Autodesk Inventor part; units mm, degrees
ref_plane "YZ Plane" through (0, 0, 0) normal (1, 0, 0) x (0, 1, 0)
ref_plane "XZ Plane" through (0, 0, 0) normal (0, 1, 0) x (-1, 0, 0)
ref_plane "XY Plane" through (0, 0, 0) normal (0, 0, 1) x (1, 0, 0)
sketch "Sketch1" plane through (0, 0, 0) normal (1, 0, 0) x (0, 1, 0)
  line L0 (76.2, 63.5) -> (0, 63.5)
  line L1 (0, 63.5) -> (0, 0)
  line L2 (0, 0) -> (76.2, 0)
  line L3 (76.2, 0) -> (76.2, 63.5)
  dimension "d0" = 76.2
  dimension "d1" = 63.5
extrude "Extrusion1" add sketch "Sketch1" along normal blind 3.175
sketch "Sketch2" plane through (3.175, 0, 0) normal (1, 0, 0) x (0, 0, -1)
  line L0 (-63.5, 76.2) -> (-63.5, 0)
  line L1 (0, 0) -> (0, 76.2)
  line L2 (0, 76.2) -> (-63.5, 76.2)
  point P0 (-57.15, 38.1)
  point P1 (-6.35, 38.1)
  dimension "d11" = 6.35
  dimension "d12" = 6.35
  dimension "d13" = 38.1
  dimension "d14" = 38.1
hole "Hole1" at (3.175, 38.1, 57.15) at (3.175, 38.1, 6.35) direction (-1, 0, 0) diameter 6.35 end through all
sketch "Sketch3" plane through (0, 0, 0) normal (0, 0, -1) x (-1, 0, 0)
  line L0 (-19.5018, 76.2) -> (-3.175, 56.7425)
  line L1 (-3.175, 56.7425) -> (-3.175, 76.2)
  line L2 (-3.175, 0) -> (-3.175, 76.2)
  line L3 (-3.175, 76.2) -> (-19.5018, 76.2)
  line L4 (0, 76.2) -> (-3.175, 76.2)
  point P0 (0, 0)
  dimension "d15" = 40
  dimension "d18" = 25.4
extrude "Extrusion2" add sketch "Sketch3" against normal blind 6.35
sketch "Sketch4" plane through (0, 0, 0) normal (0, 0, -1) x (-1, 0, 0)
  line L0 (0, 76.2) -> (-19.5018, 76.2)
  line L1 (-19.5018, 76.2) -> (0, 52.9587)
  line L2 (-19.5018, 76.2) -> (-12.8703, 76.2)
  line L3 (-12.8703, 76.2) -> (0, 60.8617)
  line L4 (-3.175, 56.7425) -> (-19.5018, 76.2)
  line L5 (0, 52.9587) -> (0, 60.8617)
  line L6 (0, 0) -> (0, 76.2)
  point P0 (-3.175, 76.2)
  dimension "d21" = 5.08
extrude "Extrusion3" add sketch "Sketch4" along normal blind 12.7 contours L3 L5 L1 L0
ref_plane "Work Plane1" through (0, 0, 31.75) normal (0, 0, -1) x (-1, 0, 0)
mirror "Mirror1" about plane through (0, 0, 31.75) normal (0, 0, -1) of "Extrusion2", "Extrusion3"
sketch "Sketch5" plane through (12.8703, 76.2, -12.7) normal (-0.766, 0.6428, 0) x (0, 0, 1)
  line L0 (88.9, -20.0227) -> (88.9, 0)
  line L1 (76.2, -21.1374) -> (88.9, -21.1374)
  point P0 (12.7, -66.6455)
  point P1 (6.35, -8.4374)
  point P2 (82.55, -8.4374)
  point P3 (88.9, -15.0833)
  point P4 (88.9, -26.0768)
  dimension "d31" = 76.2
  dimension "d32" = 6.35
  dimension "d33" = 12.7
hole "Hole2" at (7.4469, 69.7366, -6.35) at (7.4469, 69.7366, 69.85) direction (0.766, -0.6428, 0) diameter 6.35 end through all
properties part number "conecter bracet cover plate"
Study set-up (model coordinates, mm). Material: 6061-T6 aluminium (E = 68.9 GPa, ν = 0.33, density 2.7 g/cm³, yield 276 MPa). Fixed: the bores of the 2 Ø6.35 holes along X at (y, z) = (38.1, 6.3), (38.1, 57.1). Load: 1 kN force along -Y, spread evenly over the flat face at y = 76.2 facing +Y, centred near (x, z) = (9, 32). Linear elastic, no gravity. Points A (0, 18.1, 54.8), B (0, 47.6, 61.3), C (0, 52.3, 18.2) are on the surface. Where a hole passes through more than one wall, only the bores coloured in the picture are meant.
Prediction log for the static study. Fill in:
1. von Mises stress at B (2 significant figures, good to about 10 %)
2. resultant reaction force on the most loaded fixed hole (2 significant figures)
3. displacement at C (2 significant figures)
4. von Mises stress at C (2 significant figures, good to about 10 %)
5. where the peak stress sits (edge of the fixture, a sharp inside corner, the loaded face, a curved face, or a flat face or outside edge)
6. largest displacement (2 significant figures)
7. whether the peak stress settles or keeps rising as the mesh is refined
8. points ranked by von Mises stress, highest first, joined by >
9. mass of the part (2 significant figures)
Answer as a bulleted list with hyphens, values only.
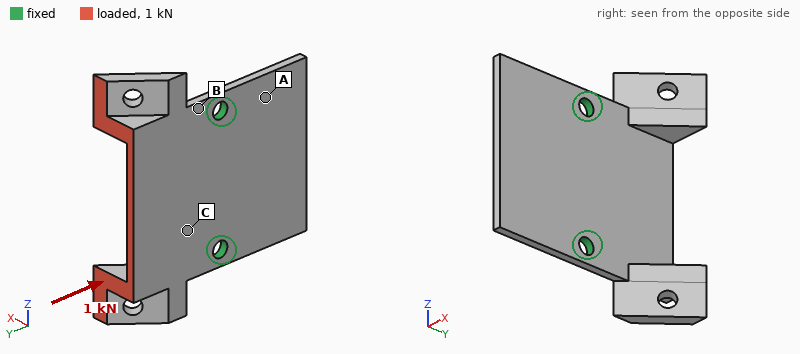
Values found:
- 91 MPa
- 500 N
- 0.087 mm
- 56 MPa
- edge of the fixture
- 0.53 mm
- keeps rising
- B > C > A
- 54 g
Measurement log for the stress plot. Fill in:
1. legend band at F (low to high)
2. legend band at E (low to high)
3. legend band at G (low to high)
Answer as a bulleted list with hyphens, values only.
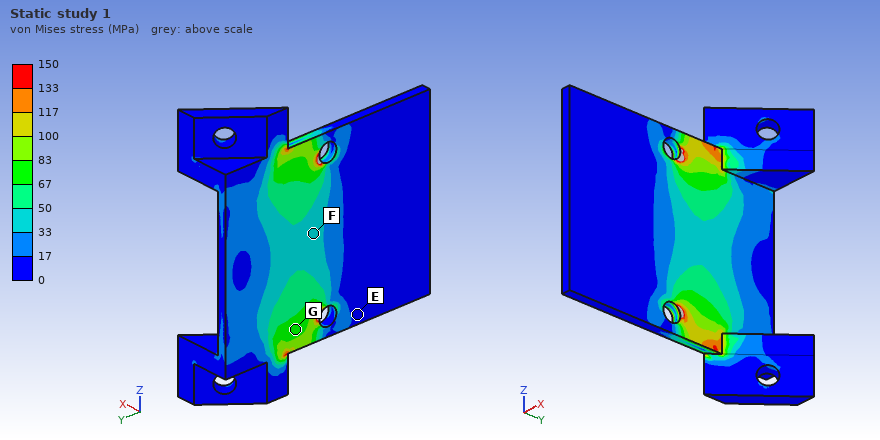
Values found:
- 33 to 50 MPa
- 0 to 17 MPa
- 67 to 83 MPa
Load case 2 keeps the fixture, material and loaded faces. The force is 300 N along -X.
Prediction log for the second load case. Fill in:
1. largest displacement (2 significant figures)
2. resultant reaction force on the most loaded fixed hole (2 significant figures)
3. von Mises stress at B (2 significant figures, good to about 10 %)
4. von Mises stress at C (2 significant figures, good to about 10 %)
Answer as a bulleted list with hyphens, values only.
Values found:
- 0.56 mm
- 150 N
- 110 MPa
- 56 MPa
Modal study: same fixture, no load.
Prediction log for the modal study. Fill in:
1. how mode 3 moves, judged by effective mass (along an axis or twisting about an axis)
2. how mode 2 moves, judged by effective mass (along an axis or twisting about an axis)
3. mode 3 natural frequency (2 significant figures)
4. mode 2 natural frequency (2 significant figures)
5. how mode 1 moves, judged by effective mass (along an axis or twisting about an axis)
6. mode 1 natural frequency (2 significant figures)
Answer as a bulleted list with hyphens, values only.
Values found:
- along X
- twisting about Y
- 1700 Hz
- 1400 Hz
- along X
- 1100 Hz
